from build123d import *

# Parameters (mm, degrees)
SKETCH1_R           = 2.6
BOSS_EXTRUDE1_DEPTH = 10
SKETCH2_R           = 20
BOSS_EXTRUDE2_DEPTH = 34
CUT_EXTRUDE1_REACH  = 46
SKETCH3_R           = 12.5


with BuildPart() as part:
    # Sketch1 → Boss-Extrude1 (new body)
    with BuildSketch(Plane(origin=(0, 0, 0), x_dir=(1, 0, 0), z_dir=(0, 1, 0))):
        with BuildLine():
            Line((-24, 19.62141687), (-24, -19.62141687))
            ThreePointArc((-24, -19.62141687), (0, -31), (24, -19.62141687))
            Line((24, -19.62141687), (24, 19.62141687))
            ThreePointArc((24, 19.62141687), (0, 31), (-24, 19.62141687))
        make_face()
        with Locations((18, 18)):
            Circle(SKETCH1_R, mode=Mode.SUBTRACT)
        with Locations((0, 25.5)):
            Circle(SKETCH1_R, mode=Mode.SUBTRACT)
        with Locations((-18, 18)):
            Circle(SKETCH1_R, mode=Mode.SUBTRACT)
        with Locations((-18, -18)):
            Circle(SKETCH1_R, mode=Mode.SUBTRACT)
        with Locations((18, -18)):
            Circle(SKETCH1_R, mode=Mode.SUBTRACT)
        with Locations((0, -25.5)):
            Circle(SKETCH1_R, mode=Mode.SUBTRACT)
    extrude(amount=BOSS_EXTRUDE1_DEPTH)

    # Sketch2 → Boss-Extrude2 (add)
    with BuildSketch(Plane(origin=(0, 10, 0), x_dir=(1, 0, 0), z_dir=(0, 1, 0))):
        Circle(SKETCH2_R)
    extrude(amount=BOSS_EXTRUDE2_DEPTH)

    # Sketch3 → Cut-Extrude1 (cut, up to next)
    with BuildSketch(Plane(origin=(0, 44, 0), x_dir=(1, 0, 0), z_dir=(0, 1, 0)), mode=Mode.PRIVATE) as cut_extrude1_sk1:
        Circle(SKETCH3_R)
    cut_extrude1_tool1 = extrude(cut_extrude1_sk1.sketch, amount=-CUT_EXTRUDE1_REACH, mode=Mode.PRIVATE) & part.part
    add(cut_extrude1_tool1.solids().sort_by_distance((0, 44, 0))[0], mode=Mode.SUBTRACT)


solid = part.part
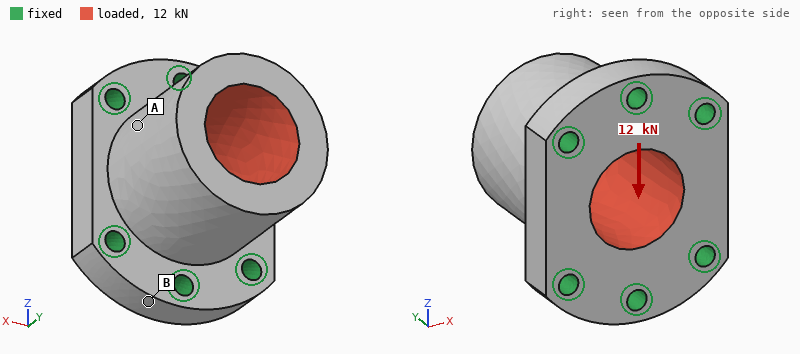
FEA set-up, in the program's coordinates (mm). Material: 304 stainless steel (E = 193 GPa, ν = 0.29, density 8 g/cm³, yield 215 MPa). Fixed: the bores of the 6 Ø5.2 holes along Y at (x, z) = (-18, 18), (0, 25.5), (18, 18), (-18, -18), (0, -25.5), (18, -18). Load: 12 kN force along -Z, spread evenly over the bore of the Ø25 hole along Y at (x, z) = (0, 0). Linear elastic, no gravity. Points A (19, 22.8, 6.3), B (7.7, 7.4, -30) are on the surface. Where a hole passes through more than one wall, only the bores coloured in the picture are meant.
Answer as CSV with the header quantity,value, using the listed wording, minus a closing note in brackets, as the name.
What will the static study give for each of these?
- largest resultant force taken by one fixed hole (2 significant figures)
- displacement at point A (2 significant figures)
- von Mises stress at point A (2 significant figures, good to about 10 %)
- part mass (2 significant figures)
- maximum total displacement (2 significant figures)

quantity,value
largest resultant force taken by one fixed hole,3.1 kN
displacement at point A,5.1 µm
von Mises stress at point A,17 MPa
part mass,370 g
maximum total displacement,12 µm
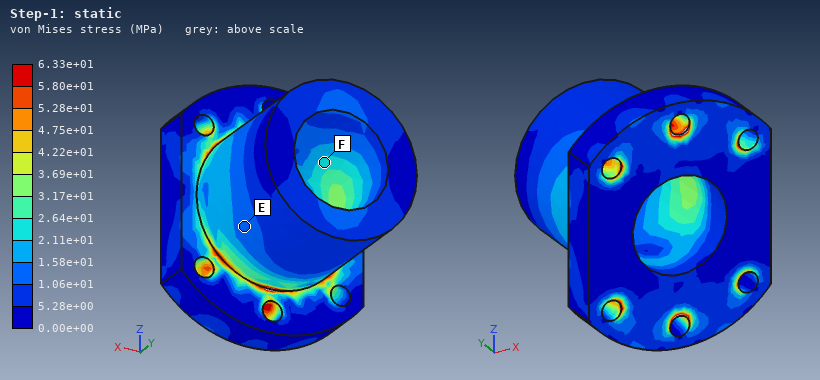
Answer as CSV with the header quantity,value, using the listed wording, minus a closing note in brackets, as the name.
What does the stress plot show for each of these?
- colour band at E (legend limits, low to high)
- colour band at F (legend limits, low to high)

quantity,value
colour band at E,1.06e+01 to 1.58e+01 MPa
colour band at F,2.11e+01 to 2.64e+01 MPa
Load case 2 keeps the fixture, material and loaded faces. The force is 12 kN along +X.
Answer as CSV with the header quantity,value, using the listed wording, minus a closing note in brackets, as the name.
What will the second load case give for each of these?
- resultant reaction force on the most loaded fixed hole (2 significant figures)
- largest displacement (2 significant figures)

quantity,value
resultant reaction force on the most loaded fixed hole,3.8 kN
largest displacement,16 µm
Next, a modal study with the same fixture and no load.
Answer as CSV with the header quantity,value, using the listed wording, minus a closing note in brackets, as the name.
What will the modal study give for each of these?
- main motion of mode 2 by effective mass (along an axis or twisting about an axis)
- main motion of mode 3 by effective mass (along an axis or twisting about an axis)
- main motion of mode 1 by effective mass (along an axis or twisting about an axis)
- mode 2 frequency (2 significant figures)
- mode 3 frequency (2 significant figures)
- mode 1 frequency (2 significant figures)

quantity,value
main motion of mode 2 by effective mass,along Z
main motion of mode 3 by effective mass,along Y
main motion of mode 1 by effective mass,along X
mode 2 frequency,11 kHz
mode 3 frequency,18 kHz
mode 1 frequency,9800 Hz
